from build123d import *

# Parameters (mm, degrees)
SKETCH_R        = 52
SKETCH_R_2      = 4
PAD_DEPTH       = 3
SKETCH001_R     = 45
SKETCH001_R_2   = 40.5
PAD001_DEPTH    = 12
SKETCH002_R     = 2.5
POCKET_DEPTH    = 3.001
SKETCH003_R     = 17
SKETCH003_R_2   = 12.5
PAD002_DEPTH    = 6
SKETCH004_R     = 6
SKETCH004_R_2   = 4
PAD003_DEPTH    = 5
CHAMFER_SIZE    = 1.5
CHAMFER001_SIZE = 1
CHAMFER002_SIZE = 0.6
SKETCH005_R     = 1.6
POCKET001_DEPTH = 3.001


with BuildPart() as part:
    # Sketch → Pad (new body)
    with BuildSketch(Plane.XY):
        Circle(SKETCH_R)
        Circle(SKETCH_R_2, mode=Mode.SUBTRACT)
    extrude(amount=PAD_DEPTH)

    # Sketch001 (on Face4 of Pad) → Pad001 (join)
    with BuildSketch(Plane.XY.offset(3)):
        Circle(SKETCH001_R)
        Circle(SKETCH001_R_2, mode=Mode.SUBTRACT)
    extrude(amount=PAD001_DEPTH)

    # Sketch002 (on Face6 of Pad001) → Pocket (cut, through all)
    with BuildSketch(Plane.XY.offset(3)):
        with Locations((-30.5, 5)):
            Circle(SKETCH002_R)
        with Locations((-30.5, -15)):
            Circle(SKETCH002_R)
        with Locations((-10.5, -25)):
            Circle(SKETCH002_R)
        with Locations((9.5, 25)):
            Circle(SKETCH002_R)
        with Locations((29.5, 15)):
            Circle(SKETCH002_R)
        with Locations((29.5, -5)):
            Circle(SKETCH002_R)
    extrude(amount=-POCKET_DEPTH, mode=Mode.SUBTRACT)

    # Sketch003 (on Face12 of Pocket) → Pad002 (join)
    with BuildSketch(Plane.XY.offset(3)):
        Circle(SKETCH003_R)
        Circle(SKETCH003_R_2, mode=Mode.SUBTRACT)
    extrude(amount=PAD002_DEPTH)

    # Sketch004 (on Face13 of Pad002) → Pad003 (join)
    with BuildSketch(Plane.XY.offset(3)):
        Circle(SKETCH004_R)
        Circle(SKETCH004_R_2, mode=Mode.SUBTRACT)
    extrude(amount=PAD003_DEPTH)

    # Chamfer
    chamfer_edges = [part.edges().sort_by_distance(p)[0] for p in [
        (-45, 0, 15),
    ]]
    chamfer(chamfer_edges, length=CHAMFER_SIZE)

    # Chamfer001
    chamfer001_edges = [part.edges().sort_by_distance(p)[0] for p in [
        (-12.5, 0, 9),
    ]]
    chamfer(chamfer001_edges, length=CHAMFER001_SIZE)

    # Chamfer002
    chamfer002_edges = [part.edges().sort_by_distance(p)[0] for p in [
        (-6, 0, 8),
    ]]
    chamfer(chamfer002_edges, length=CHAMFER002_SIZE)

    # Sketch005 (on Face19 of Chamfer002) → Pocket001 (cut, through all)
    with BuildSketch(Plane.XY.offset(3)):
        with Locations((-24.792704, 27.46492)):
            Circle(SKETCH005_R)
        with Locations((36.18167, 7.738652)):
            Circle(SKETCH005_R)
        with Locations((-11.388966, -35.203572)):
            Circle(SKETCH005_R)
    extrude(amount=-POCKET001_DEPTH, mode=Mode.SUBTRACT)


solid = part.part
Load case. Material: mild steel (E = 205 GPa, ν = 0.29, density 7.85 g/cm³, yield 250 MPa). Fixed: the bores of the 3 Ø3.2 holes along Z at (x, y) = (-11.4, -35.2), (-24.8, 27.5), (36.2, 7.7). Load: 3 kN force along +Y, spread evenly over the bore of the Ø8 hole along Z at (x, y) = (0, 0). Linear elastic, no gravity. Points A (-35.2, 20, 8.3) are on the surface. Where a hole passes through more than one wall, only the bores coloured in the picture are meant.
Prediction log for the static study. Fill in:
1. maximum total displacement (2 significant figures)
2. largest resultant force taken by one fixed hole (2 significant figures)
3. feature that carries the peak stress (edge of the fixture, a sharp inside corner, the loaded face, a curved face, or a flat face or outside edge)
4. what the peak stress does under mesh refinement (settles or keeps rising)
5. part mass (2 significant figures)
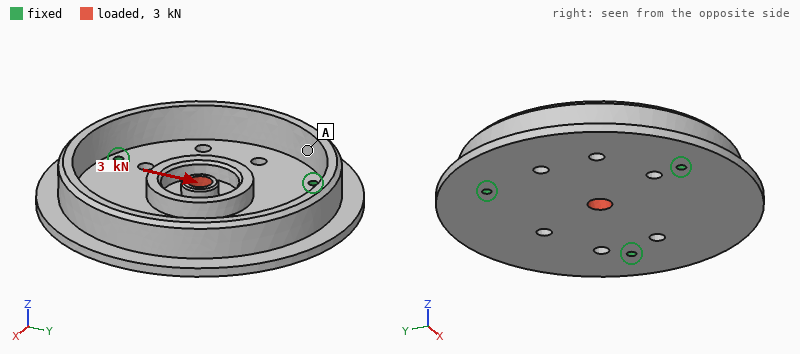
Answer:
14 µm
1.1 kN
edge of the fixture
keeps rising
330 g
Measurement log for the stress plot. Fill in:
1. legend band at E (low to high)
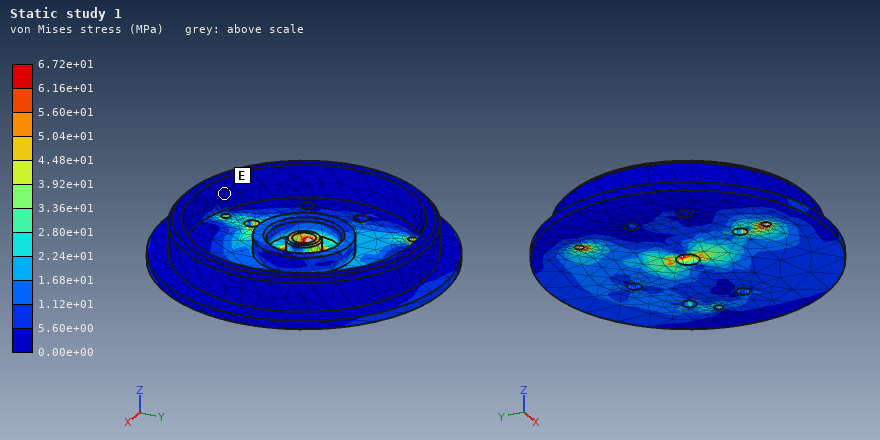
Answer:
0.00e+00 to 5.60e+00 MPa
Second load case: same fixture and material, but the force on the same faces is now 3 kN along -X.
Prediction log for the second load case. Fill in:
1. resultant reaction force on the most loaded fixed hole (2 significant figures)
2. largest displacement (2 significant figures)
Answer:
1.1 kN
14 µm
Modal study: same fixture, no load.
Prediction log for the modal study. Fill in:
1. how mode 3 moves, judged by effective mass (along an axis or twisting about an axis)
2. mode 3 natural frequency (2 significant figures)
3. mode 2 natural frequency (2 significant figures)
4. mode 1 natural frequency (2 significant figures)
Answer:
along Z
4400 Hz
2700 Hz
2700 Hz
